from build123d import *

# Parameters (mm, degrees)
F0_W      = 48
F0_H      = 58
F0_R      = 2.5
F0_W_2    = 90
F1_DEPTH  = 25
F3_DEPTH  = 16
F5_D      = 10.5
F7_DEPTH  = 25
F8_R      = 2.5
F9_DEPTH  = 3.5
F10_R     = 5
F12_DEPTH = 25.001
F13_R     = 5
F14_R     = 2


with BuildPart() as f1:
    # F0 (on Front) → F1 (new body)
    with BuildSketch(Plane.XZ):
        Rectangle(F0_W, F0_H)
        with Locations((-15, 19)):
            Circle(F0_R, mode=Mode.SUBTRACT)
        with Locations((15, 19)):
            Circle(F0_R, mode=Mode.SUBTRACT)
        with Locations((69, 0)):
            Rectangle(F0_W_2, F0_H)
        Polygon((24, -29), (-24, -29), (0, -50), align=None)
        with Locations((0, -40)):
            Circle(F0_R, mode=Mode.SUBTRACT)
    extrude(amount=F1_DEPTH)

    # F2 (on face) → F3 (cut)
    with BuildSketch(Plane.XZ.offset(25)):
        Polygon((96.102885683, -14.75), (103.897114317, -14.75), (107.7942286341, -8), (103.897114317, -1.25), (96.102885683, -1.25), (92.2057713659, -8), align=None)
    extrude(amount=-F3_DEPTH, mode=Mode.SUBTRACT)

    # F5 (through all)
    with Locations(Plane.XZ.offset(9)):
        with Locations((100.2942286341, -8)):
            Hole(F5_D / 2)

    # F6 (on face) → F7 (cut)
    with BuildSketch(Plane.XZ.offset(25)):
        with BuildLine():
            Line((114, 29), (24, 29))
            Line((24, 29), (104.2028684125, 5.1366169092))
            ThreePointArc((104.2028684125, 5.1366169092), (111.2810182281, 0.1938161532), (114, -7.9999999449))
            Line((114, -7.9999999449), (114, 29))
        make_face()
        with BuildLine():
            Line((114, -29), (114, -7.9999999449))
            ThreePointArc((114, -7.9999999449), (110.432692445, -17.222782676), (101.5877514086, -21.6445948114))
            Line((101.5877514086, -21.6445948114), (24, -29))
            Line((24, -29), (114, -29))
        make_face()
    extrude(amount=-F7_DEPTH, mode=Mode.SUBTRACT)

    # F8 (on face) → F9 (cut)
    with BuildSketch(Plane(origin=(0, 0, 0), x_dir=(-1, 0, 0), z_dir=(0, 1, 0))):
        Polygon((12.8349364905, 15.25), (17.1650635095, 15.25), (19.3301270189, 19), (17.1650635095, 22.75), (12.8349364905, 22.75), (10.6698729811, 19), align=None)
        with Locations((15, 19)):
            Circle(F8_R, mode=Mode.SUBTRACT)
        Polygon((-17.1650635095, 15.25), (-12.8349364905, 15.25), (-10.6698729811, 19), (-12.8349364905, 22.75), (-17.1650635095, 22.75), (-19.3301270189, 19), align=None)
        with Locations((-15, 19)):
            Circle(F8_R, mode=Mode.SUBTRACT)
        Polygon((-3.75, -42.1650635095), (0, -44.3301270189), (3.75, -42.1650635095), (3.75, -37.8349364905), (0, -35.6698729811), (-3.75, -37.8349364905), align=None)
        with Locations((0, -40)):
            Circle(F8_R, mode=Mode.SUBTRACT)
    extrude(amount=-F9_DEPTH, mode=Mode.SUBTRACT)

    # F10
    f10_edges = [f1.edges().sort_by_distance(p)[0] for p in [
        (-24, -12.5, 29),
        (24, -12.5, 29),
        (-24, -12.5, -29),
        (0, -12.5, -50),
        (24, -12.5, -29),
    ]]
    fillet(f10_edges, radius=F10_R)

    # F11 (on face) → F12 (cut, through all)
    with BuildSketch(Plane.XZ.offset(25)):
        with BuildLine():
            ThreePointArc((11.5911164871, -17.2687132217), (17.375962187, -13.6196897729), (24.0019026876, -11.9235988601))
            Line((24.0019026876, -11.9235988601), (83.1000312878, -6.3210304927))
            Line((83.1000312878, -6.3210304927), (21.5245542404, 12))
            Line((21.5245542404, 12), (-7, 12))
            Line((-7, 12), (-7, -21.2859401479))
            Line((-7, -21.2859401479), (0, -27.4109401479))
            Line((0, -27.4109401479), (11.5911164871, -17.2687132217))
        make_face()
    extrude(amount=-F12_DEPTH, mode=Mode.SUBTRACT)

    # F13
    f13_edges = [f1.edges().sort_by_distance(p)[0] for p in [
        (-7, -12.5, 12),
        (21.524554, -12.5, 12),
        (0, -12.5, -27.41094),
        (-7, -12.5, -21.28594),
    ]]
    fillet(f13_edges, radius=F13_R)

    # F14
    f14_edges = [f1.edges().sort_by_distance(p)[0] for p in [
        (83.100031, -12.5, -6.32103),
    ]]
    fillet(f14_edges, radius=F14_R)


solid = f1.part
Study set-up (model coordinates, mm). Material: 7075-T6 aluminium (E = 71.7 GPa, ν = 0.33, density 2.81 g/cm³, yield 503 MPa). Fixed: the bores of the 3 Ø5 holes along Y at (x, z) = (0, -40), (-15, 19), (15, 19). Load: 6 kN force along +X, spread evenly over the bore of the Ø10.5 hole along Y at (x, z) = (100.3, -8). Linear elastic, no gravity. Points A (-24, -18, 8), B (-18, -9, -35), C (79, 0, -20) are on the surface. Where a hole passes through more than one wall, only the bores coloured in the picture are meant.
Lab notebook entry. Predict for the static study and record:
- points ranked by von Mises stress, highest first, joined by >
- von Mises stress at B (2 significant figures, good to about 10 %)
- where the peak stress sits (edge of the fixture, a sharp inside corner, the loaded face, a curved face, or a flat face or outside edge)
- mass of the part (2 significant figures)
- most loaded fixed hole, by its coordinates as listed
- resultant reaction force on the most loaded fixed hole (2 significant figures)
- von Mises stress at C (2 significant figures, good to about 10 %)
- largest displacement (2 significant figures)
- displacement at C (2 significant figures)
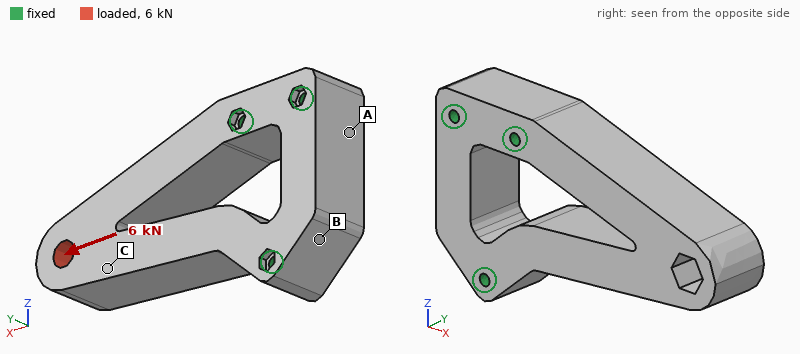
C > B > A
8.8 MPa
edge of the fixture
350 g
(0, -40)
3.3 kN
23 MPa
0.11 mm
0.061 mm
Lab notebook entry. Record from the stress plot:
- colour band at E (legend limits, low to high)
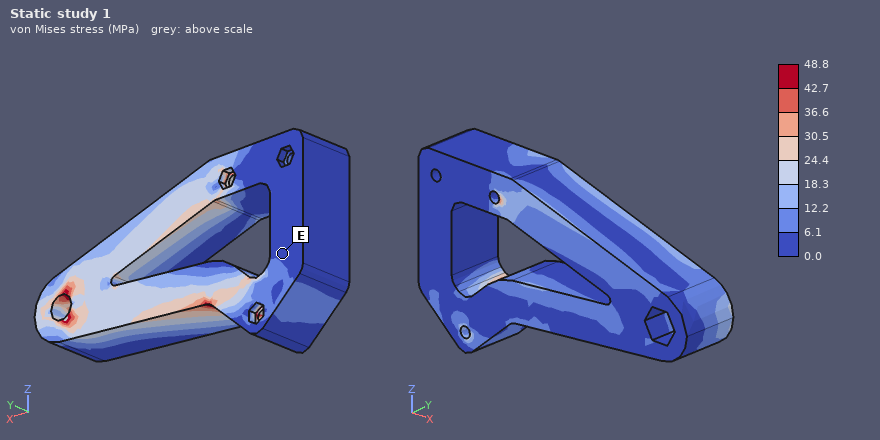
0.0 to 6.1 MPa
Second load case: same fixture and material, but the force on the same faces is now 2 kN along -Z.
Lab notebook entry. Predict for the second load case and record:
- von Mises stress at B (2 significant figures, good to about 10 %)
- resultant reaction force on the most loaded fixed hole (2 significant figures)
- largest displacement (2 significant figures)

4.5 MPa
3.0 kN
60 µm
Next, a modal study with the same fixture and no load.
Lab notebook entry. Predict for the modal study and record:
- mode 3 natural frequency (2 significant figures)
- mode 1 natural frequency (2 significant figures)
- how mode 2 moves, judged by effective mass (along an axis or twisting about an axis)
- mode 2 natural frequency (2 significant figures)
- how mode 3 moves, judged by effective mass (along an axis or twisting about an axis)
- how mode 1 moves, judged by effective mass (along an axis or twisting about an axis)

5900 Hz
1800 Hz
along Z
3700 Hz
along X
along Y
